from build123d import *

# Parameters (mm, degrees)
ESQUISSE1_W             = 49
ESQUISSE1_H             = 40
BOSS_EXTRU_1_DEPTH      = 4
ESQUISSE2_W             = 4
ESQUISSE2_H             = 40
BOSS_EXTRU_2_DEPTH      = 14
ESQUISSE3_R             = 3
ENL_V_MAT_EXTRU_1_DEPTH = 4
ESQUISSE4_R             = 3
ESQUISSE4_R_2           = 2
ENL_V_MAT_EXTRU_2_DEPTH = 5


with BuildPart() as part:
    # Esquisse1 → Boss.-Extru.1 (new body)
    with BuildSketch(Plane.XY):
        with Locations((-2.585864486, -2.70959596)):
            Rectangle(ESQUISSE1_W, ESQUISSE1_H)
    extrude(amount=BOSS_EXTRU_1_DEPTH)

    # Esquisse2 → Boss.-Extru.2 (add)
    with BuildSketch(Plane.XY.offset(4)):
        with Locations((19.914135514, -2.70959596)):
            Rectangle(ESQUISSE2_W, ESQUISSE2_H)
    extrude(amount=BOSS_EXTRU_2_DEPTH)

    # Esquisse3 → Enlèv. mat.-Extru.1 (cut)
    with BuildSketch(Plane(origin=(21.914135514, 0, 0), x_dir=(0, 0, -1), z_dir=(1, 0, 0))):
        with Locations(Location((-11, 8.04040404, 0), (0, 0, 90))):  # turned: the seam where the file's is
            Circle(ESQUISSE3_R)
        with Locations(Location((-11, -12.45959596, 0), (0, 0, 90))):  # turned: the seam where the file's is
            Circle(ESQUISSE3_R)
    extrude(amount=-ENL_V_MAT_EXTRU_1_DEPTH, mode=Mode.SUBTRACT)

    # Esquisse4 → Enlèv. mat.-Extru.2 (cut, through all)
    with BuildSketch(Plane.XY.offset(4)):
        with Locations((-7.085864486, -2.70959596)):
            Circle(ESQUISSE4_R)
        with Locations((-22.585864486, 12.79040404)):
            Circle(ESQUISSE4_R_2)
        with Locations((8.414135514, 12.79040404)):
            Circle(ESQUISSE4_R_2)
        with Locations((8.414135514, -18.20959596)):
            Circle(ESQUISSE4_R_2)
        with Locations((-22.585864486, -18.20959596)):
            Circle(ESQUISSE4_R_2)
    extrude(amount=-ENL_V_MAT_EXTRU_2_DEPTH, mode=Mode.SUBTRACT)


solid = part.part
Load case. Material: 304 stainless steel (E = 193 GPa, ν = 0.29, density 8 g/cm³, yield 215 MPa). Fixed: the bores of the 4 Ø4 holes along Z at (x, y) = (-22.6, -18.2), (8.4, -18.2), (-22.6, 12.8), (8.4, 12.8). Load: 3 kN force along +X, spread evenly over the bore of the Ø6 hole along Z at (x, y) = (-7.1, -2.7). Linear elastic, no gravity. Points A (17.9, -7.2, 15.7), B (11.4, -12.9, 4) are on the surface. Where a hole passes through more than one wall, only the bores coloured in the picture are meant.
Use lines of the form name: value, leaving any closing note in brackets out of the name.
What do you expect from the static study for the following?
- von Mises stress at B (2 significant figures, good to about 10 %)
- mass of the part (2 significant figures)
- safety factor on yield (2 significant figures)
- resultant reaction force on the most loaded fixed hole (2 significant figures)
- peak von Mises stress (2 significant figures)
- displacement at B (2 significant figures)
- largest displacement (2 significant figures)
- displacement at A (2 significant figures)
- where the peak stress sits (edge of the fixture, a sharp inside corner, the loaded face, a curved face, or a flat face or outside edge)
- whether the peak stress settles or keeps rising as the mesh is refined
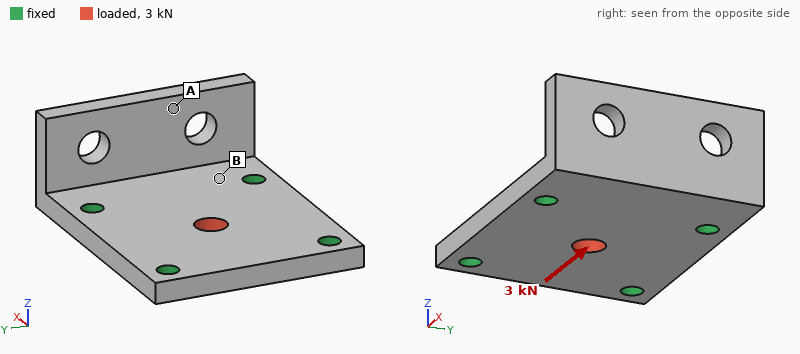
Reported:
von Mises stress at B: 12 MPa
mass of the part: 76 g
safety factor on yield: 3.1
resultant reaction force on the most loaded fixed hole: 850 N
peak von Mises stress: 69 MPa
displacement at B: 0.61 µm
largest displacement: 2.8 µm
displacement at A: 0.98 µm
where the peak stress sits: the loaded face
whether the peak stress settles or keeps rising as the mesh is refined: settles
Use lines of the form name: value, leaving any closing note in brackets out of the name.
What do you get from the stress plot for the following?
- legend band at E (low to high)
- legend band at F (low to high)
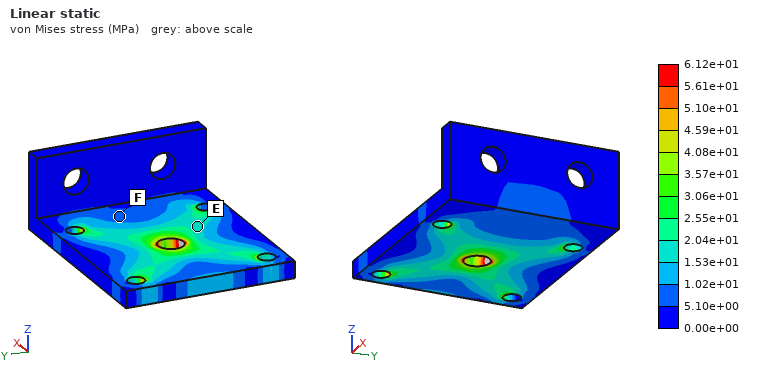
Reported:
legend band at E: 1.53e+01 to 2.04e+01 MPa
legend band at F: 5.10e+00 to 1.02e+01 MPa
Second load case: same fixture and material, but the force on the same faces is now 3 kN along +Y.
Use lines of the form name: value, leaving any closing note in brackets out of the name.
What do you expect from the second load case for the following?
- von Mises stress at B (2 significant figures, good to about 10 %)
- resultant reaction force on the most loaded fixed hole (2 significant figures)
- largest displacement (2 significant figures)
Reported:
von Mises stress at B: 5.8 MPa
resultant reaction force on the most loaded fixed hole: 850 N
largest displacement: 2.9 µm
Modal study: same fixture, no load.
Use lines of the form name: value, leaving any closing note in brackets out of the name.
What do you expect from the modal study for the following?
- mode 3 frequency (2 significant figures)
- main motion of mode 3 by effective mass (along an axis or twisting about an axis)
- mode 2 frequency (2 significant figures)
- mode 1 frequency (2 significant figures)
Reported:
mode 3 frequency: 14 kHz
main motion of mode 3 by effective mass: along Z
mode 2 frequency: 9600 Hz
mode 1 frequency: 5600 Hz
